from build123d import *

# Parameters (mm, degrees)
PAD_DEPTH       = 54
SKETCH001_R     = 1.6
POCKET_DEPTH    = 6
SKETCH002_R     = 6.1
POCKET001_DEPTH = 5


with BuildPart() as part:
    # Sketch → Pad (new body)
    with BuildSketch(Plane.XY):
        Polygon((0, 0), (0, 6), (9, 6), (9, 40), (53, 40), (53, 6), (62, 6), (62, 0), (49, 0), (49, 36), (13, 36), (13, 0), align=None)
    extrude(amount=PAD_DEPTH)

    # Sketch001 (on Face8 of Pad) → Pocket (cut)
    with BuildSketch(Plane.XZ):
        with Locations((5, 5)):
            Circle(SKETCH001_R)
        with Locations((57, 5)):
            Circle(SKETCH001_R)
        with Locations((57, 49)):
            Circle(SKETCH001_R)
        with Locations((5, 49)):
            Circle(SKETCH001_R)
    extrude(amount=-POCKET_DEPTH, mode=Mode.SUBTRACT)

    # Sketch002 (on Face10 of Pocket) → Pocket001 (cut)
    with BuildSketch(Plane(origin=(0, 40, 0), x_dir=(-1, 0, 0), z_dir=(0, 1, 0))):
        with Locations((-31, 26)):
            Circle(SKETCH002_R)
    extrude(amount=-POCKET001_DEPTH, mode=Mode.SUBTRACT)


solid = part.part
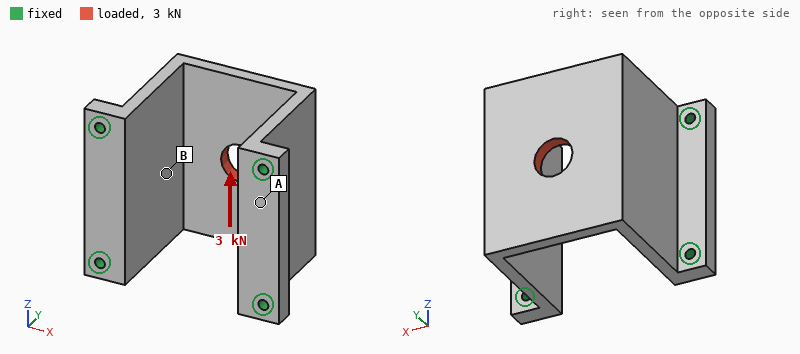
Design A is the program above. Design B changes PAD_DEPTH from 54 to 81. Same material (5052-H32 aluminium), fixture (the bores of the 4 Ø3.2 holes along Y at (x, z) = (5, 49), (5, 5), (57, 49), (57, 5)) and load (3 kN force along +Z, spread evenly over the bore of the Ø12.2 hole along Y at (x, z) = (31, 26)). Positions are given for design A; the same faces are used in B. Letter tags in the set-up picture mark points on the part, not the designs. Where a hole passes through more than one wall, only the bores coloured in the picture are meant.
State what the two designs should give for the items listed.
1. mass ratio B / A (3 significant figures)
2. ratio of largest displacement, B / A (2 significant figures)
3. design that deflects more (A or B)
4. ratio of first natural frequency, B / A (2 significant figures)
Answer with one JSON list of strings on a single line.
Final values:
["1.51", "1.1", "B", "0.96"]
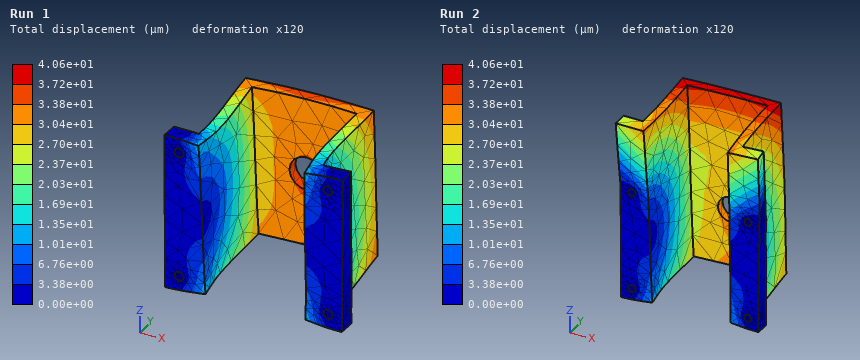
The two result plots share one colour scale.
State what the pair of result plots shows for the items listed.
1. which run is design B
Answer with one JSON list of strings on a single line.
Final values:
["Run 2"]
